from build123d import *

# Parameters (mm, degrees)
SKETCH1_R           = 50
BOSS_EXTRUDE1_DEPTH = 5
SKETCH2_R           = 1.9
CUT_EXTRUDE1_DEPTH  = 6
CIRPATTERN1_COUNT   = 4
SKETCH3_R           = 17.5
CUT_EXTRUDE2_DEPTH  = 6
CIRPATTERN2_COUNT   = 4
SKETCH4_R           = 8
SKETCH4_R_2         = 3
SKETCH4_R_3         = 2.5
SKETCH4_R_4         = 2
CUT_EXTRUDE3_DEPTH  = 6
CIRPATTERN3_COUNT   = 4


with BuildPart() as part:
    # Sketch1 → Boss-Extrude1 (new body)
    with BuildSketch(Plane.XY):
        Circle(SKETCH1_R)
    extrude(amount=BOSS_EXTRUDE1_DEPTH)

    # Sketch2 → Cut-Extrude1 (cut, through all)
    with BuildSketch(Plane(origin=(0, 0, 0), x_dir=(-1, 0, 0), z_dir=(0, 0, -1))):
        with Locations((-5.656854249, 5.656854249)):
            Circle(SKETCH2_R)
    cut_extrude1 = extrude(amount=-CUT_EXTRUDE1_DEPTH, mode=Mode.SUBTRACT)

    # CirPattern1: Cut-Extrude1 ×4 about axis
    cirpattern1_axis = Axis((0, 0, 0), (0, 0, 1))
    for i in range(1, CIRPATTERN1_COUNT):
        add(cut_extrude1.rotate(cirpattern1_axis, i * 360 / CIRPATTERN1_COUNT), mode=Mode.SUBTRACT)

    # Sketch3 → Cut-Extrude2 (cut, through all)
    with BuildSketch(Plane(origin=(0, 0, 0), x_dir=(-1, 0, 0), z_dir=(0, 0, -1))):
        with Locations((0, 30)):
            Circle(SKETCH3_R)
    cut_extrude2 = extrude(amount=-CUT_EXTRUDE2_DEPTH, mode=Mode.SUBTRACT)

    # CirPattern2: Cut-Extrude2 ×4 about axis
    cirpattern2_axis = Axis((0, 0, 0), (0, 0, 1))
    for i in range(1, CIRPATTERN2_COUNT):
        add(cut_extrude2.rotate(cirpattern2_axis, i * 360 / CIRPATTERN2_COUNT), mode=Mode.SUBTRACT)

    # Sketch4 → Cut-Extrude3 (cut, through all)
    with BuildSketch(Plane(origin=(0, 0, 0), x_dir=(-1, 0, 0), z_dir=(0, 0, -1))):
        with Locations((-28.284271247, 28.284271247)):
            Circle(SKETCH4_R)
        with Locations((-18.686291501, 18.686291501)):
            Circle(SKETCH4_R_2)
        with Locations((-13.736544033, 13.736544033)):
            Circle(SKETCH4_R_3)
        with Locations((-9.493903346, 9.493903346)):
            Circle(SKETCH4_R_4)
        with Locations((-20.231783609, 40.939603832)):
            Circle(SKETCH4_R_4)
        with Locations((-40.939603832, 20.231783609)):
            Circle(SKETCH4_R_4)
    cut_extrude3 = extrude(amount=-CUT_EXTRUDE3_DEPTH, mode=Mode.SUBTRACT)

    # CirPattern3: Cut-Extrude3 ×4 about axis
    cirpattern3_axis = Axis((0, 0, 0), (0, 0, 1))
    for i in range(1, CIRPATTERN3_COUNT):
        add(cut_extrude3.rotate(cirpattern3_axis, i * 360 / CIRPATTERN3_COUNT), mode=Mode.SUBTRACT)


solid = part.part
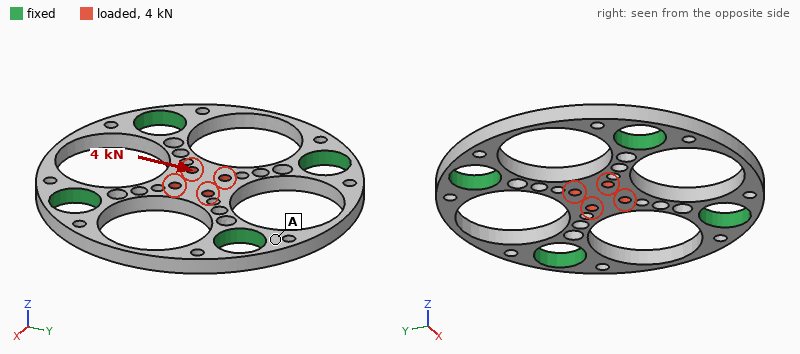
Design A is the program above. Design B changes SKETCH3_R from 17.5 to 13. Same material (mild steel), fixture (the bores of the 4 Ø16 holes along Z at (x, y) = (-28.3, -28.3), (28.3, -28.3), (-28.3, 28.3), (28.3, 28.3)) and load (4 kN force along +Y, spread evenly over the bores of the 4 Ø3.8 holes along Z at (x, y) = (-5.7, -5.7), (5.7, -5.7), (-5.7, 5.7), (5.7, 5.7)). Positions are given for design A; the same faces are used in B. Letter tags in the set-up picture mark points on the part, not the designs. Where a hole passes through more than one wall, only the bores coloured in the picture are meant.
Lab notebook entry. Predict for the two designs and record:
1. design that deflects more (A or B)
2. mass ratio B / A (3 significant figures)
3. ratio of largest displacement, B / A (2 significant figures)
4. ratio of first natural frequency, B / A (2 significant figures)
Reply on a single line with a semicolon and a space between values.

A; 1.61; 0.36; 1.2
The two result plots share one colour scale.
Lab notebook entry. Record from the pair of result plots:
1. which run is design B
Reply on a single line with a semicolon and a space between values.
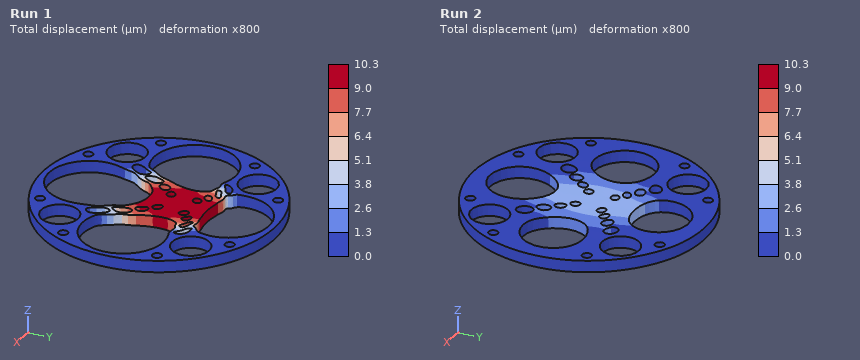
Run 2
